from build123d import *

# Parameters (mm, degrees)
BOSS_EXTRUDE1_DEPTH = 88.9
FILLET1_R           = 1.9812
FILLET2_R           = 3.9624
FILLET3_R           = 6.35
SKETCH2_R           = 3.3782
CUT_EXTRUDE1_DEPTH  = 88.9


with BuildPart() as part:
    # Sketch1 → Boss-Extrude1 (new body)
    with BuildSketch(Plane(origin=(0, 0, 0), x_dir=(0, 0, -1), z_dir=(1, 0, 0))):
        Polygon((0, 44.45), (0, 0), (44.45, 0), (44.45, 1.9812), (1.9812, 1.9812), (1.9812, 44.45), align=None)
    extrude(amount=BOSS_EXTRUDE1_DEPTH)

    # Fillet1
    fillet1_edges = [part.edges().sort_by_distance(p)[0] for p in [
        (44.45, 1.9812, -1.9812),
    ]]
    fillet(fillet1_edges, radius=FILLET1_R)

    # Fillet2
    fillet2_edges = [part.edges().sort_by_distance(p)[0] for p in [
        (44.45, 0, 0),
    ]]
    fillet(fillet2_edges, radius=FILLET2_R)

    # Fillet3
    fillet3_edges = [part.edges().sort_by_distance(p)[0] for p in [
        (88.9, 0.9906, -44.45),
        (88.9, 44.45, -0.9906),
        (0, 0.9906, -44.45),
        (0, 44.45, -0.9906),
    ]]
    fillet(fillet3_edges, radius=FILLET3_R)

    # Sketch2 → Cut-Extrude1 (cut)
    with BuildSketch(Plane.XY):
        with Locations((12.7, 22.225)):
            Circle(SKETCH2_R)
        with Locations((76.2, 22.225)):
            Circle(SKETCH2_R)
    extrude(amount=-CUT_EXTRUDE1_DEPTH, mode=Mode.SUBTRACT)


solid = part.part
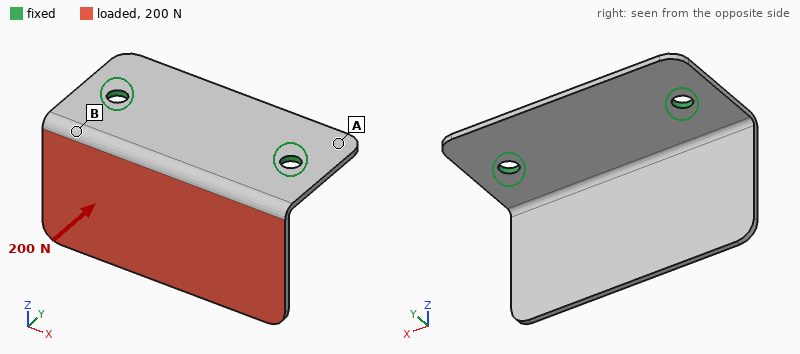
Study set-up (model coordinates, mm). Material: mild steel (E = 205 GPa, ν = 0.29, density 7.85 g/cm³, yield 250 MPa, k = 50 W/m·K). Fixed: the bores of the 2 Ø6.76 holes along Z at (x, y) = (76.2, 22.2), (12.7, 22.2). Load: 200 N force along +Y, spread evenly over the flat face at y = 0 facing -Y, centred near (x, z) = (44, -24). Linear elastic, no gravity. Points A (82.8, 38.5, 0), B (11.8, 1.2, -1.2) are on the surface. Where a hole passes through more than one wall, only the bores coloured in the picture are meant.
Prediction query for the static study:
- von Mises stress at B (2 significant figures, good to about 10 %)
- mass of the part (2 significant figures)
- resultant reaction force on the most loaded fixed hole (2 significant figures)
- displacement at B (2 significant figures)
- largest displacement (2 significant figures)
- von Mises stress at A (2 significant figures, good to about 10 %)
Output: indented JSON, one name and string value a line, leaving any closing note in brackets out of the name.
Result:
{
  "von Mises stress at B": "53 MPa",
  "mass of the part": "120 g",
  "resultant reaction force on the most loaded fixed hole": "100 N",
  "displacement at B": "0.085 mm",
  "largest displacement": "0.51 mm",
  "von Mises stress at A": "12 MPa"
}
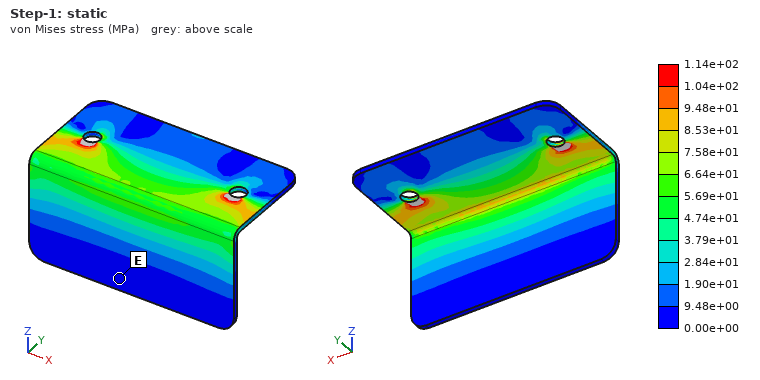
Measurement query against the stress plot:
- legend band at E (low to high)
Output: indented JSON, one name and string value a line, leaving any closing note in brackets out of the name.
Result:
{
  "legend band at E": "0.00e+00 to 9.48e+00 MPa"
}
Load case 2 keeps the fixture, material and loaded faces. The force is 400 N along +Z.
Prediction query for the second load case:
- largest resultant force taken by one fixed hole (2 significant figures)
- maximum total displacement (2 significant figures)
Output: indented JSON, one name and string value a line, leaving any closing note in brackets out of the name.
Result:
{
  "largest resultant force taken by one fixed hole": "200 N",
  "maximum total displacement": "0.40 mm"
}
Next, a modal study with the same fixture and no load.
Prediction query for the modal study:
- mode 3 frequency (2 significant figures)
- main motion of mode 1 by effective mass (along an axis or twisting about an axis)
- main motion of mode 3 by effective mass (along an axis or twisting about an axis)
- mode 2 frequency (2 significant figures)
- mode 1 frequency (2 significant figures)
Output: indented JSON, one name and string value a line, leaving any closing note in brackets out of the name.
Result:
{
  "mode 3 frequency": "1600 Hz",
  "main motion of mode 1 by effective mass": "along Y",
  "main motion of mode 3 by effective mass": "along Z",
  "mode 2 frequency": "960 Hz",
  "mode 1 frequency": "500 Hz"
}
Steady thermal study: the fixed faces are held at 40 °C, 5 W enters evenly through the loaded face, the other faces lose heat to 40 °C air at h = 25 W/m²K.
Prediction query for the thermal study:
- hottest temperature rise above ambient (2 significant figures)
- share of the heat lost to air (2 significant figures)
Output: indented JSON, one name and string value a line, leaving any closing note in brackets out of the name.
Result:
{
  "hottest temperature rise above ambient": "18 K",
  "share of the heat lost to air": "46 %"
}
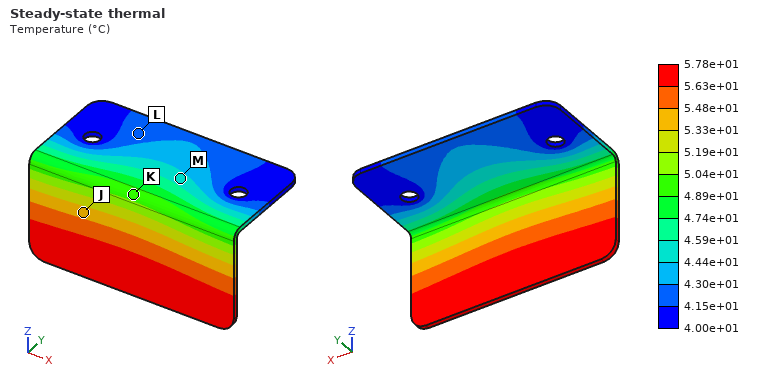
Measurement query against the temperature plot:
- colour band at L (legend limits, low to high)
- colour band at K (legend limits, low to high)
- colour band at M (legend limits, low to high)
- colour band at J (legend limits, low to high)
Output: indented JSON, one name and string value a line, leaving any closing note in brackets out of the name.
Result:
{
  "colour band at L": "4.15e+01 to 4.30e+01 °C",
  "colour band at K": "4.89e+01 to 5.04e+01 °C",
  "colour band at M": "4.44e+01 to 4.59e+01 °C",
  "colour band at J": "5.33e+01 to 5.48e+01 °C"
}
